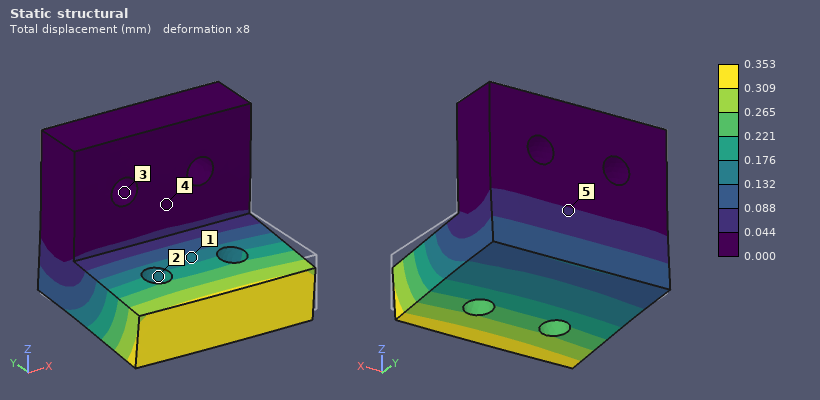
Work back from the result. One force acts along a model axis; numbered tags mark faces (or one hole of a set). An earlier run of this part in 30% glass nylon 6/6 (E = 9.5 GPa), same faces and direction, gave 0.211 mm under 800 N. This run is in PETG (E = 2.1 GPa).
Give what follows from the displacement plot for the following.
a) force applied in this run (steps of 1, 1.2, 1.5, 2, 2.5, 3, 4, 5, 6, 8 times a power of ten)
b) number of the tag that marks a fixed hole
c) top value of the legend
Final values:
300 N
3
0.353 mm
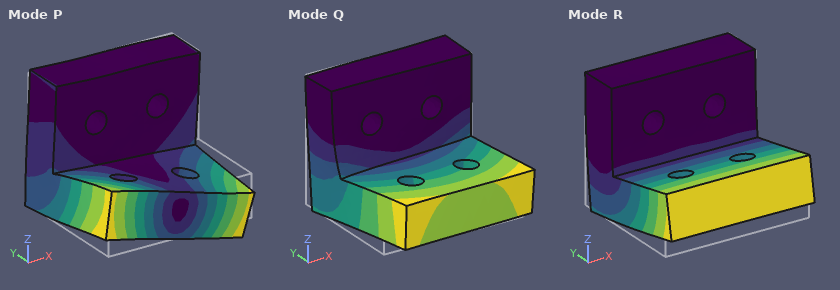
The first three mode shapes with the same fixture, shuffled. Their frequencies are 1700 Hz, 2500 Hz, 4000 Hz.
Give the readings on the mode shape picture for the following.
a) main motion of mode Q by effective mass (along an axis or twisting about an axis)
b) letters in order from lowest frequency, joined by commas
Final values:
along X
R, Q, P
